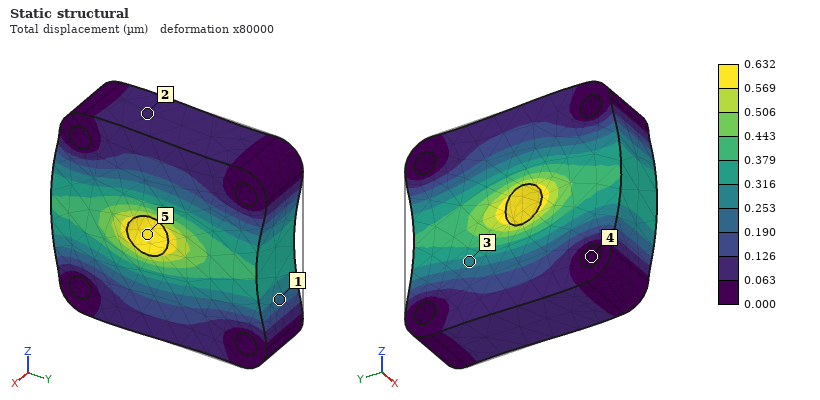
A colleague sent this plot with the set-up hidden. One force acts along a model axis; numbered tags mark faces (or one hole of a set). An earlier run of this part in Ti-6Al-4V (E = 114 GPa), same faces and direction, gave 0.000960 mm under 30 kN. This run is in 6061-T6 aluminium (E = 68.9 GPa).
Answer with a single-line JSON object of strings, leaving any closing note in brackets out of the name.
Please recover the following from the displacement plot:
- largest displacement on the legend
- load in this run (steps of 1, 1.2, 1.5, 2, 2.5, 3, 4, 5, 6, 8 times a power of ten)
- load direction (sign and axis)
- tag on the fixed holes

{"largest displacement on the legend": "0.632 µm", "load in this run": "12 kN", "load direction": "-Y", "tag on the fixed holes": "4"}
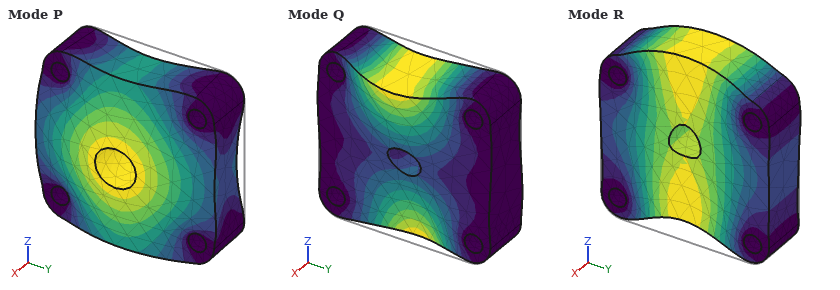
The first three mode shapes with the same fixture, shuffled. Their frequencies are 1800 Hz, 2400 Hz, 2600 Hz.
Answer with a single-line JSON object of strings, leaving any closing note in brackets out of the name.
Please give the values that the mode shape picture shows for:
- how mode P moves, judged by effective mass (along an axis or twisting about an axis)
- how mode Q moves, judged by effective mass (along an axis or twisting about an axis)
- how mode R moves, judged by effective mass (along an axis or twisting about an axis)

{"how mode P moves, judged by effective mass": "along X", "how mode Q moves, judged by effective mass": "twisting about Y", "how mode R moves, judged by effective mass": "along Z"}
